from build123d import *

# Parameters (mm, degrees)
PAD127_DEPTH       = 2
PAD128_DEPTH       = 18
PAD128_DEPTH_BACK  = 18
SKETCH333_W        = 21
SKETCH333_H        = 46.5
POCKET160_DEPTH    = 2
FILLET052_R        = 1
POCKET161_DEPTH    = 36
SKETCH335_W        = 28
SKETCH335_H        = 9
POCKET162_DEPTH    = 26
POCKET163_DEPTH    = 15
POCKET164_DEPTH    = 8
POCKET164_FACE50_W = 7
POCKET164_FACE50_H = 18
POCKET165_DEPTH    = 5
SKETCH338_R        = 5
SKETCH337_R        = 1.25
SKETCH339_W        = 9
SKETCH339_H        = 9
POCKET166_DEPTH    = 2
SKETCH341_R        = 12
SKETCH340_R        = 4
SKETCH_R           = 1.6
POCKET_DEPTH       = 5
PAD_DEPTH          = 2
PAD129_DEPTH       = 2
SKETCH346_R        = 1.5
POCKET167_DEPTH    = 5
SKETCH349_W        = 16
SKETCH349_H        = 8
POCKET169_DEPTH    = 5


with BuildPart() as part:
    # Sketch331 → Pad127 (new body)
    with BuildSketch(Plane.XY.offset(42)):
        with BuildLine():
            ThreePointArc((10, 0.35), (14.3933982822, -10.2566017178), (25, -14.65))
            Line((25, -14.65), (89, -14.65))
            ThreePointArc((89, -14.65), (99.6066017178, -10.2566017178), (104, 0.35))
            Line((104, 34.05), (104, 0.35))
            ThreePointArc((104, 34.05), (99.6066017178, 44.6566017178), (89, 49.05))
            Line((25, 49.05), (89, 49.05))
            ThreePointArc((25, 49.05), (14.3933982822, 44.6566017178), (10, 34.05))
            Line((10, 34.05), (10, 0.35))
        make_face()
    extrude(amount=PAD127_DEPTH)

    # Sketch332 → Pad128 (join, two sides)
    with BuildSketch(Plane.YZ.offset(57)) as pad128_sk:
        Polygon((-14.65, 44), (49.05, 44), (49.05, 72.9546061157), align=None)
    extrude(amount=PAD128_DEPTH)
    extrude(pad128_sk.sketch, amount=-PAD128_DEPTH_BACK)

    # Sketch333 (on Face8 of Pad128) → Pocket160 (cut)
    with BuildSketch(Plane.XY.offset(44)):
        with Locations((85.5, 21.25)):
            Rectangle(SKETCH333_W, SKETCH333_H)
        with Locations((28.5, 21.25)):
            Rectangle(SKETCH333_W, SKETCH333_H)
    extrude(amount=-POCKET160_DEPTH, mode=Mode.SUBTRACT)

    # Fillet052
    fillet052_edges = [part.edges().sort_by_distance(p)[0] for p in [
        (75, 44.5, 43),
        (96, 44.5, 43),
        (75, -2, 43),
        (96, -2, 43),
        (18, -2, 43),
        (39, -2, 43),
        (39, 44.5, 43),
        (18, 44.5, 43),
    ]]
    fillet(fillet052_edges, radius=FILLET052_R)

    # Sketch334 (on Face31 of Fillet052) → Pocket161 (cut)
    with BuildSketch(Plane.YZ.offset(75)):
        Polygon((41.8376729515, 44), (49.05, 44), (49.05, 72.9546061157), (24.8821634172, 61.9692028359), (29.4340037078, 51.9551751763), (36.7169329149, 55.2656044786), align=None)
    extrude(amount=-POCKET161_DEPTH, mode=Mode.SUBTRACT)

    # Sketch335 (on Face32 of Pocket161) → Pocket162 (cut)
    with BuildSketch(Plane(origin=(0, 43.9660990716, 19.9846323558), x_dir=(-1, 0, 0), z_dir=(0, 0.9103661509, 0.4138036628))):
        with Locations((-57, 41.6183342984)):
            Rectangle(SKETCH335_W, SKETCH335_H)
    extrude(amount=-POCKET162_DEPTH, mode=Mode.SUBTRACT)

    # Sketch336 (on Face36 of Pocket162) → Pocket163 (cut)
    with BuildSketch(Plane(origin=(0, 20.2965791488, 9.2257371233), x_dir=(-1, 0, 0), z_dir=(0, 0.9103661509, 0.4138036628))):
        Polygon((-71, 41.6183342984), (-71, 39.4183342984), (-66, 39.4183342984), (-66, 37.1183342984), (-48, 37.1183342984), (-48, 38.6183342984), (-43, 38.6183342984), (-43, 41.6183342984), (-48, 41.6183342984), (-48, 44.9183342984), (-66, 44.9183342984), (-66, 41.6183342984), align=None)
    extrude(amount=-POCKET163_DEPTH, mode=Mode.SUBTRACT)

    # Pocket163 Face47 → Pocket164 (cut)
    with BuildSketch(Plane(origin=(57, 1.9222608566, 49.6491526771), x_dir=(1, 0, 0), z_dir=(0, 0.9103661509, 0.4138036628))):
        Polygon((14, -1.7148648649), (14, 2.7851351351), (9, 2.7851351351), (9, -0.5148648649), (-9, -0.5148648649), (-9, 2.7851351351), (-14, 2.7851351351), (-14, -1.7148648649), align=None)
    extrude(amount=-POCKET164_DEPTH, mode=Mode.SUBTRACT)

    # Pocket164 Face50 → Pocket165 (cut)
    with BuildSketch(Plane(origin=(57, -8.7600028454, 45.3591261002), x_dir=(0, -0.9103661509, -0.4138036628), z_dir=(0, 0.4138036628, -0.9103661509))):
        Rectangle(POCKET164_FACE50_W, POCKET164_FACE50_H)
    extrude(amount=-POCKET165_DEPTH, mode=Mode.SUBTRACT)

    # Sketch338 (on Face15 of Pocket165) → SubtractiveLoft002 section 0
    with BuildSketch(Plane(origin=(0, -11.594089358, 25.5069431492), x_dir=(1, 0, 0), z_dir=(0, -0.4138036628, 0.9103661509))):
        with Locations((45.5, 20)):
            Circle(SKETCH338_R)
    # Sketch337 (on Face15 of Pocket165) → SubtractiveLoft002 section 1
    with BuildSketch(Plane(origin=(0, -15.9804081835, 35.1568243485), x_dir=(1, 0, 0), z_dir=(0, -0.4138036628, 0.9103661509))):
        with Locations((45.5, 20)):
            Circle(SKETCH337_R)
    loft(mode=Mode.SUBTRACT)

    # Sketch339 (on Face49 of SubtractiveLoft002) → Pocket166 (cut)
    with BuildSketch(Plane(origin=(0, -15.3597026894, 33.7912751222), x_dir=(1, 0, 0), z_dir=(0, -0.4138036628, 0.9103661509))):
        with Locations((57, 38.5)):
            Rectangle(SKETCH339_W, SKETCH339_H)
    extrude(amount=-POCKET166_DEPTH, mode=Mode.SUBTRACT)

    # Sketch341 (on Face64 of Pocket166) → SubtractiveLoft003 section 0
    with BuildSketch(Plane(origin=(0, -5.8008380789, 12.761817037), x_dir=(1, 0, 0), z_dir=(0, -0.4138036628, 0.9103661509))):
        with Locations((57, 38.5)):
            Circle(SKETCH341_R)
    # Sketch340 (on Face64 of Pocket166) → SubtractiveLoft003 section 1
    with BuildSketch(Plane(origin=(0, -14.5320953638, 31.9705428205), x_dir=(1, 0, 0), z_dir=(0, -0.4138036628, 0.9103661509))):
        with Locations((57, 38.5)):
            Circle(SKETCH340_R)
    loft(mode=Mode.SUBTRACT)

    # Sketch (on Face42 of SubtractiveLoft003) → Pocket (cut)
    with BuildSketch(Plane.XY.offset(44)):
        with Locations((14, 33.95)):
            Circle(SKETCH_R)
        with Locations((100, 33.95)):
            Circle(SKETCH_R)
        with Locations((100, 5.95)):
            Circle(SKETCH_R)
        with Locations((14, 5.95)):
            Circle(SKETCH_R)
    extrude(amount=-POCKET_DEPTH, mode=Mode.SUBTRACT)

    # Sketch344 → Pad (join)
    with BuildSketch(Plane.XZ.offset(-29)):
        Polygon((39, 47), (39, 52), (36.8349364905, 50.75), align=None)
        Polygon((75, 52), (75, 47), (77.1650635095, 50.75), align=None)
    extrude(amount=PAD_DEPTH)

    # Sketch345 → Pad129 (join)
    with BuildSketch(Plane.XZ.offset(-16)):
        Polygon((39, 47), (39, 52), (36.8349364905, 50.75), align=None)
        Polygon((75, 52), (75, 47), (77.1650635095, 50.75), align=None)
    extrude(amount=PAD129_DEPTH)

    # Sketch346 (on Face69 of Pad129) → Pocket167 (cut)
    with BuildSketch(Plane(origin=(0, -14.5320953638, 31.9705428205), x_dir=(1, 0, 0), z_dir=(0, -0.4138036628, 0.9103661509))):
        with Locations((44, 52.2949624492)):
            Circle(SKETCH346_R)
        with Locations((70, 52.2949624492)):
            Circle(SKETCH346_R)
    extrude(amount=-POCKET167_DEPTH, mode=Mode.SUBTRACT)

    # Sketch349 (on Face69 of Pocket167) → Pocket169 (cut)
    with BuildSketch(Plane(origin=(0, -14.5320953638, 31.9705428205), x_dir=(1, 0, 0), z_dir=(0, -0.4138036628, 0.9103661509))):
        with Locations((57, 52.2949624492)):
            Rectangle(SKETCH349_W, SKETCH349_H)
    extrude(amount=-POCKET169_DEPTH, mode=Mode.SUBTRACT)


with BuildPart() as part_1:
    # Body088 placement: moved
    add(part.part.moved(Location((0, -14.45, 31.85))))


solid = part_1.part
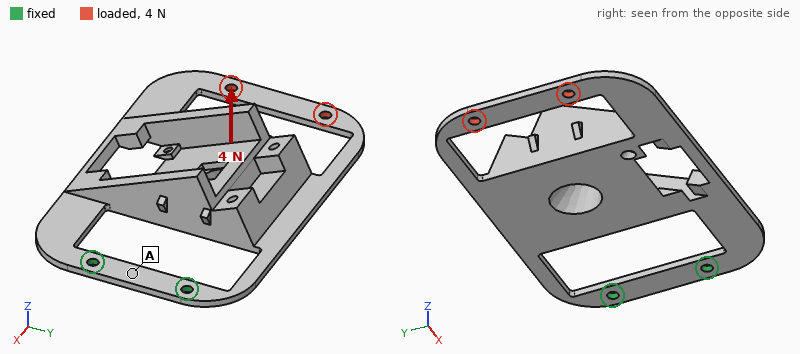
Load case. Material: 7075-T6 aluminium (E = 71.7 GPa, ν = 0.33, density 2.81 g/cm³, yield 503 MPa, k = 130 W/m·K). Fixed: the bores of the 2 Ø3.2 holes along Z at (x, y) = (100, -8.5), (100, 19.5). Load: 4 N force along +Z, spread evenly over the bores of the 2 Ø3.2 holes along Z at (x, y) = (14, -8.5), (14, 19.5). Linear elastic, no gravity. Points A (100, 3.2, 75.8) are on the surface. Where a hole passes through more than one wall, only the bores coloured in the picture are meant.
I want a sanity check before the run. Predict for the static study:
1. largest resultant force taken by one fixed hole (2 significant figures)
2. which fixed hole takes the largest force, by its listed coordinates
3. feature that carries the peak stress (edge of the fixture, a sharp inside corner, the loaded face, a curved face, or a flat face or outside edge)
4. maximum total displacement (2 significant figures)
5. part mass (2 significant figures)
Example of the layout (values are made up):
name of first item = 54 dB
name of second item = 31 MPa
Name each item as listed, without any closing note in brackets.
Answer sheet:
largest resultant force taken by one fixed hole = 2.2 N
which fixed hole takes the largest force, by its listed coordinates = (100, -8.5)
feature that carries the peak stress = a curved face
maximum total displacement = 1.2 mm
part mass = 44 g
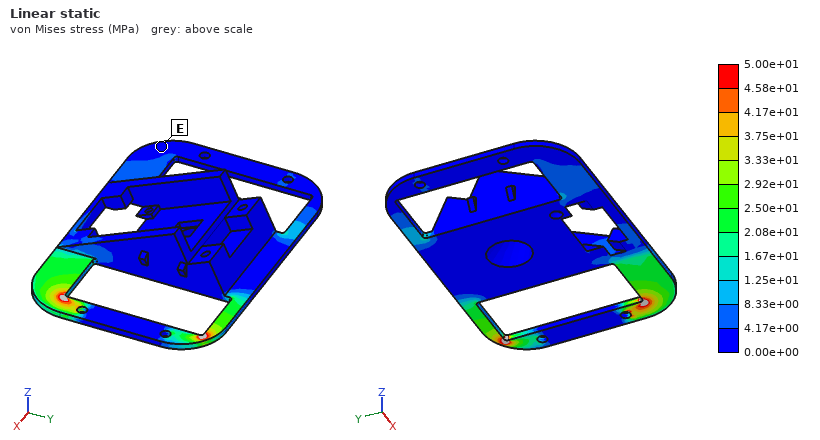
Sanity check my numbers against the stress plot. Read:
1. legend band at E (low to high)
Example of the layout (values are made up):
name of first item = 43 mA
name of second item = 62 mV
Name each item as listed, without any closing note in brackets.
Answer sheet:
legend band at E = 0.00e+00 to 4.17e+00 MPa
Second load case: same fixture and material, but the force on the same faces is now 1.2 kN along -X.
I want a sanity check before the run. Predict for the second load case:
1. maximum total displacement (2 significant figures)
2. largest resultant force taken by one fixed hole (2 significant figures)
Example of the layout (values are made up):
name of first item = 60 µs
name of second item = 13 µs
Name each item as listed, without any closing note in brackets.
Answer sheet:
maximum total displacement = 0.37 mm
largest resultant force taken by one fixed hole = 630 N
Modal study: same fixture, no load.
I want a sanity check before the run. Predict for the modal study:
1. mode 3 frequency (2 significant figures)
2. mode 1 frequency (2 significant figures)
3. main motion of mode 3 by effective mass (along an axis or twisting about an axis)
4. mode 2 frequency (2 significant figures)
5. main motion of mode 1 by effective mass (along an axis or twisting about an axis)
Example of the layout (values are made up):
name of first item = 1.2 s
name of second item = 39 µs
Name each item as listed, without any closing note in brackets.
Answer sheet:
mode 3 frequency = 790 Hz
mode 1 frequency = 91 Hz
main motion of mode 3 by effective mass = along Y
mode 2 frequency = 510 Hz
main motion of mode 1 by effective mass = along Z
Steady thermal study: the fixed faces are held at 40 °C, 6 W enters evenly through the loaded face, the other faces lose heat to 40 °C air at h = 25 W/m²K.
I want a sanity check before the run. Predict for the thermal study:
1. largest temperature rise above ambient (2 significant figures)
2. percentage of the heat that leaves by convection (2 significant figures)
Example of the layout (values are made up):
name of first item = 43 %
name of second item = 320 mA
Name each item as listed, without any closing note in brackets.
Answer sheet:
largest temperature rise above ambient = 67 K
percentage of the heat that leaves by convection = 80 %
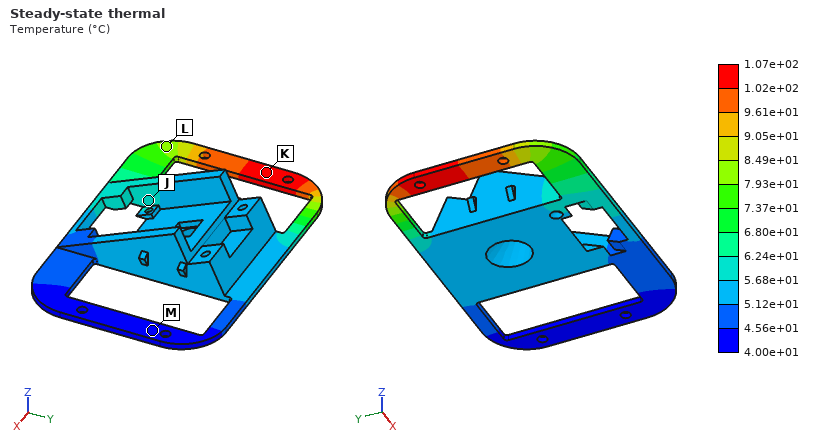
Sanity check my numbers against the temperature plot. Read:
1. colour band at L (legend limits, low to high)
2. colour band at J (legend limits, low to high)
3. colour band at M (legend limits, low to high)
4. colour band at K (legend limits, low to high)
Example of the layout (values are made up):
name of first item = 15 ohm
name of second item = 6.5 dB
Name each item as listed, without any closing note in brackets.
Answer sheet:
colour band at L = 7.93e+01 to 8.49e+01 °C
colour band at J = 5.68e+01 to 6.24e+01 °C
colour band at M = 4.00e+01 to 4.56e+01 °C
colour band at K = 1.02e+02 to 1.07e+02 °C
